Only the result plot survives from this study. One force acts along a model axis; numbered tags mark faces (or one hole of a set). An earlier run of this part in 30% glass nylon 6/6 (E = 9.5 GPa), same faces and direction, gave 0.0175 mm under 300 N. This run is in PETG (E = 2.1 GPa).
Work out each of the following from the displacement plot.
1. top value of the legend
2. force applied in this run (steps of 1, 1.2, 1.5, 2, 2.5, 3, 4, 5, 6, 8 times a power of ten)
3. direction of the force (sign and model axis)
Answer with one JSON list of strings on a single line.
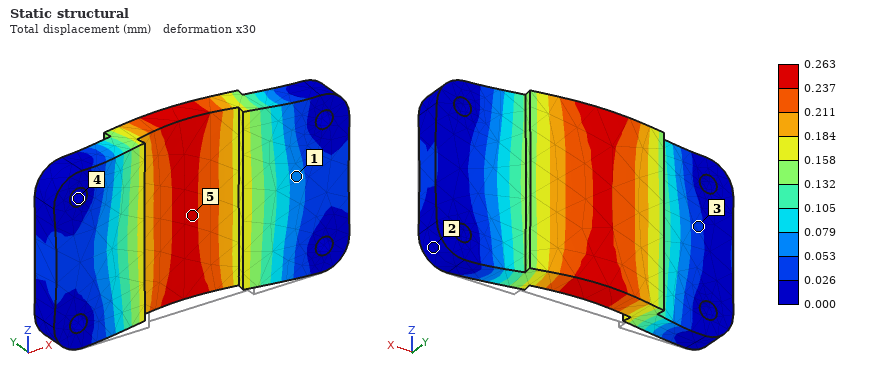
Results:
["0.263 mm", "1 kN", "+Y"]
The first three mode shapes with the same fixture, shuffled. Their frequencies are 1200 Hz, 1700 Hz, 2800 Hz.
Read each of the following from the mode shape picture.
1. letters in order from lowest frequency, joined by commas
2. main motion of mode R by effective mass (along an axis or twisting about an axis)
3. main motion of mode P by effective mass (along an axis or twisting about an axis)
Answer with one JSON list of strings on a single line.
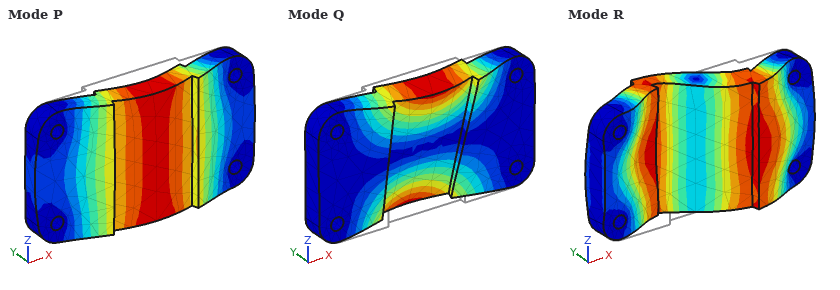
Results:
["P, Q, R", "twisting about Z", "along Y"]
